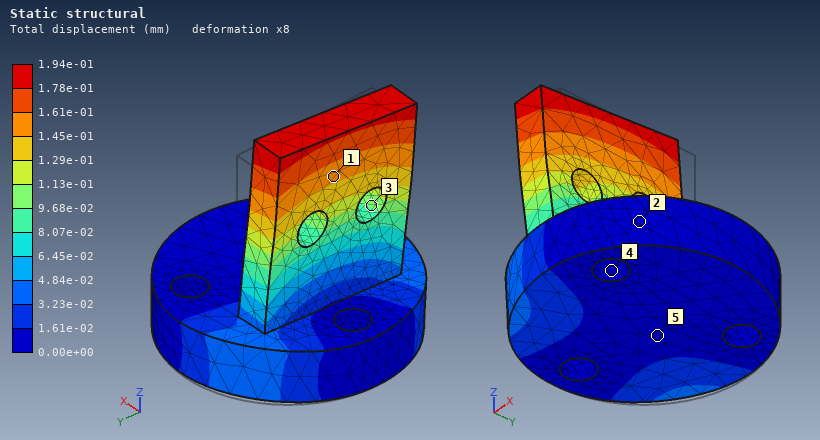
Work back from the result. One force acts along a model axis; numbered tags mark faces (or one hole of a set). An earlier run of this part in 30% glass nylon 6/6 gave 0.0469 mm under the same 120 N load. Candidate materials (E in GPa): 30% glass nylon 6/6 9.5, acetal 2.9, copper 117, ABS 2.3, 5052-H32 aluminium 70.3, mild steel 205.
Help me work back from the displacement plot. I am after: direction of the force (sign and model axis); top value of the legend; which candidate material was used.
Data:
-Y
1.94e-01 mm
ABS
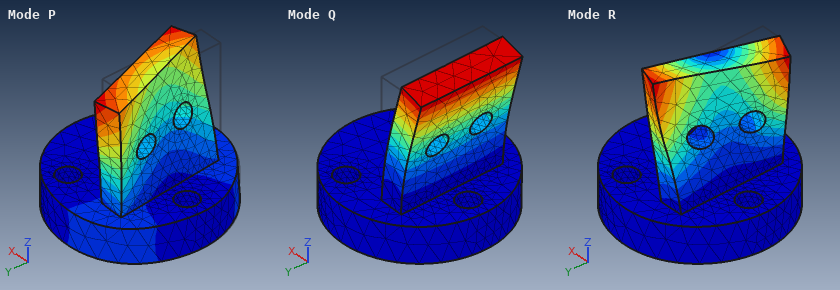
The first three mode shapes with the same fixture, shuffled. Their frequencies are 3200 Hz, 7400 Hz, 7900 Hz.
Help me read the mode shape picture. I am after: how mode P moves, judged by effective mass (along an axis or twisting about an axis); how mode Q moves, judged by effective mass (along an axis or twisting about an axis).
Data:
along Y
along X
